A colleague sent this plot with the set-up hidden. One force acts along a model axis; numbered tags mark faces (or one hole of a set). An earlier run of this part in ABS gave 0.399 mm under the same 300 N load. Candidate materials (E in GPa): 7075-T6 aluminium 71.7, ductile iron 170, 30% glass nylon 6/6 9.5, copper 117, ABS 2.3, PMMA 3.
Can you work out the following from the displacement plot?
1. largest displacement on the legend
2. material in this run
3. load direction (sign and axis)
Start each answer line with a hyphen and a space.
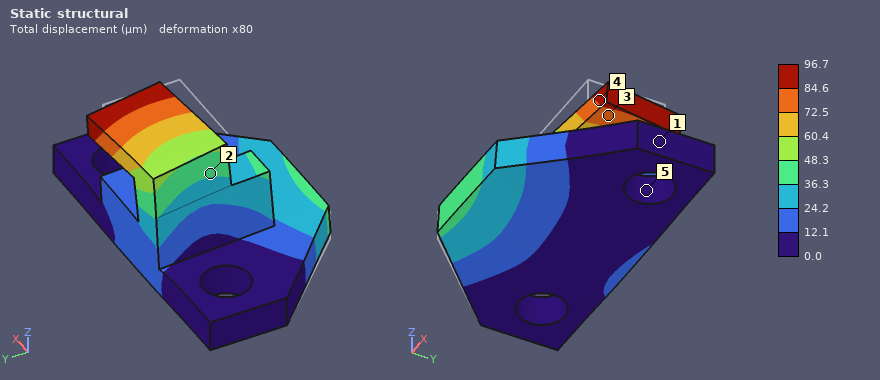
- 96.7 µm
- 30% glass nylon 6/6
- +Y
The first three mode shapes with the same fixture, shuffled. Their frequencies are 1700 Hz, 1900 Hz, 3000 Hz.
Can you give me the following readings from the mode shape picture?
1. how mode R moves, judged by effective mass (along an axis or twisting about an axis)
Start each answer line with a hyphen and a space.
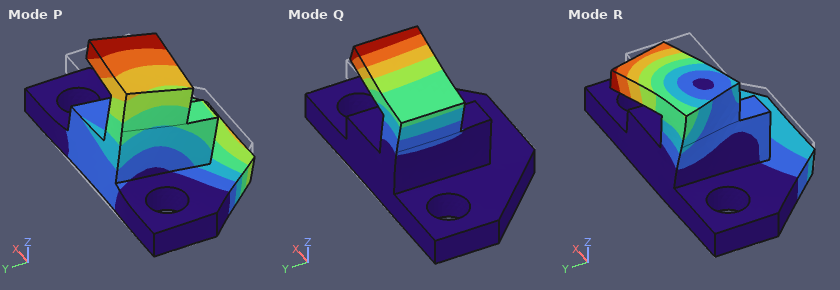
- along Z
